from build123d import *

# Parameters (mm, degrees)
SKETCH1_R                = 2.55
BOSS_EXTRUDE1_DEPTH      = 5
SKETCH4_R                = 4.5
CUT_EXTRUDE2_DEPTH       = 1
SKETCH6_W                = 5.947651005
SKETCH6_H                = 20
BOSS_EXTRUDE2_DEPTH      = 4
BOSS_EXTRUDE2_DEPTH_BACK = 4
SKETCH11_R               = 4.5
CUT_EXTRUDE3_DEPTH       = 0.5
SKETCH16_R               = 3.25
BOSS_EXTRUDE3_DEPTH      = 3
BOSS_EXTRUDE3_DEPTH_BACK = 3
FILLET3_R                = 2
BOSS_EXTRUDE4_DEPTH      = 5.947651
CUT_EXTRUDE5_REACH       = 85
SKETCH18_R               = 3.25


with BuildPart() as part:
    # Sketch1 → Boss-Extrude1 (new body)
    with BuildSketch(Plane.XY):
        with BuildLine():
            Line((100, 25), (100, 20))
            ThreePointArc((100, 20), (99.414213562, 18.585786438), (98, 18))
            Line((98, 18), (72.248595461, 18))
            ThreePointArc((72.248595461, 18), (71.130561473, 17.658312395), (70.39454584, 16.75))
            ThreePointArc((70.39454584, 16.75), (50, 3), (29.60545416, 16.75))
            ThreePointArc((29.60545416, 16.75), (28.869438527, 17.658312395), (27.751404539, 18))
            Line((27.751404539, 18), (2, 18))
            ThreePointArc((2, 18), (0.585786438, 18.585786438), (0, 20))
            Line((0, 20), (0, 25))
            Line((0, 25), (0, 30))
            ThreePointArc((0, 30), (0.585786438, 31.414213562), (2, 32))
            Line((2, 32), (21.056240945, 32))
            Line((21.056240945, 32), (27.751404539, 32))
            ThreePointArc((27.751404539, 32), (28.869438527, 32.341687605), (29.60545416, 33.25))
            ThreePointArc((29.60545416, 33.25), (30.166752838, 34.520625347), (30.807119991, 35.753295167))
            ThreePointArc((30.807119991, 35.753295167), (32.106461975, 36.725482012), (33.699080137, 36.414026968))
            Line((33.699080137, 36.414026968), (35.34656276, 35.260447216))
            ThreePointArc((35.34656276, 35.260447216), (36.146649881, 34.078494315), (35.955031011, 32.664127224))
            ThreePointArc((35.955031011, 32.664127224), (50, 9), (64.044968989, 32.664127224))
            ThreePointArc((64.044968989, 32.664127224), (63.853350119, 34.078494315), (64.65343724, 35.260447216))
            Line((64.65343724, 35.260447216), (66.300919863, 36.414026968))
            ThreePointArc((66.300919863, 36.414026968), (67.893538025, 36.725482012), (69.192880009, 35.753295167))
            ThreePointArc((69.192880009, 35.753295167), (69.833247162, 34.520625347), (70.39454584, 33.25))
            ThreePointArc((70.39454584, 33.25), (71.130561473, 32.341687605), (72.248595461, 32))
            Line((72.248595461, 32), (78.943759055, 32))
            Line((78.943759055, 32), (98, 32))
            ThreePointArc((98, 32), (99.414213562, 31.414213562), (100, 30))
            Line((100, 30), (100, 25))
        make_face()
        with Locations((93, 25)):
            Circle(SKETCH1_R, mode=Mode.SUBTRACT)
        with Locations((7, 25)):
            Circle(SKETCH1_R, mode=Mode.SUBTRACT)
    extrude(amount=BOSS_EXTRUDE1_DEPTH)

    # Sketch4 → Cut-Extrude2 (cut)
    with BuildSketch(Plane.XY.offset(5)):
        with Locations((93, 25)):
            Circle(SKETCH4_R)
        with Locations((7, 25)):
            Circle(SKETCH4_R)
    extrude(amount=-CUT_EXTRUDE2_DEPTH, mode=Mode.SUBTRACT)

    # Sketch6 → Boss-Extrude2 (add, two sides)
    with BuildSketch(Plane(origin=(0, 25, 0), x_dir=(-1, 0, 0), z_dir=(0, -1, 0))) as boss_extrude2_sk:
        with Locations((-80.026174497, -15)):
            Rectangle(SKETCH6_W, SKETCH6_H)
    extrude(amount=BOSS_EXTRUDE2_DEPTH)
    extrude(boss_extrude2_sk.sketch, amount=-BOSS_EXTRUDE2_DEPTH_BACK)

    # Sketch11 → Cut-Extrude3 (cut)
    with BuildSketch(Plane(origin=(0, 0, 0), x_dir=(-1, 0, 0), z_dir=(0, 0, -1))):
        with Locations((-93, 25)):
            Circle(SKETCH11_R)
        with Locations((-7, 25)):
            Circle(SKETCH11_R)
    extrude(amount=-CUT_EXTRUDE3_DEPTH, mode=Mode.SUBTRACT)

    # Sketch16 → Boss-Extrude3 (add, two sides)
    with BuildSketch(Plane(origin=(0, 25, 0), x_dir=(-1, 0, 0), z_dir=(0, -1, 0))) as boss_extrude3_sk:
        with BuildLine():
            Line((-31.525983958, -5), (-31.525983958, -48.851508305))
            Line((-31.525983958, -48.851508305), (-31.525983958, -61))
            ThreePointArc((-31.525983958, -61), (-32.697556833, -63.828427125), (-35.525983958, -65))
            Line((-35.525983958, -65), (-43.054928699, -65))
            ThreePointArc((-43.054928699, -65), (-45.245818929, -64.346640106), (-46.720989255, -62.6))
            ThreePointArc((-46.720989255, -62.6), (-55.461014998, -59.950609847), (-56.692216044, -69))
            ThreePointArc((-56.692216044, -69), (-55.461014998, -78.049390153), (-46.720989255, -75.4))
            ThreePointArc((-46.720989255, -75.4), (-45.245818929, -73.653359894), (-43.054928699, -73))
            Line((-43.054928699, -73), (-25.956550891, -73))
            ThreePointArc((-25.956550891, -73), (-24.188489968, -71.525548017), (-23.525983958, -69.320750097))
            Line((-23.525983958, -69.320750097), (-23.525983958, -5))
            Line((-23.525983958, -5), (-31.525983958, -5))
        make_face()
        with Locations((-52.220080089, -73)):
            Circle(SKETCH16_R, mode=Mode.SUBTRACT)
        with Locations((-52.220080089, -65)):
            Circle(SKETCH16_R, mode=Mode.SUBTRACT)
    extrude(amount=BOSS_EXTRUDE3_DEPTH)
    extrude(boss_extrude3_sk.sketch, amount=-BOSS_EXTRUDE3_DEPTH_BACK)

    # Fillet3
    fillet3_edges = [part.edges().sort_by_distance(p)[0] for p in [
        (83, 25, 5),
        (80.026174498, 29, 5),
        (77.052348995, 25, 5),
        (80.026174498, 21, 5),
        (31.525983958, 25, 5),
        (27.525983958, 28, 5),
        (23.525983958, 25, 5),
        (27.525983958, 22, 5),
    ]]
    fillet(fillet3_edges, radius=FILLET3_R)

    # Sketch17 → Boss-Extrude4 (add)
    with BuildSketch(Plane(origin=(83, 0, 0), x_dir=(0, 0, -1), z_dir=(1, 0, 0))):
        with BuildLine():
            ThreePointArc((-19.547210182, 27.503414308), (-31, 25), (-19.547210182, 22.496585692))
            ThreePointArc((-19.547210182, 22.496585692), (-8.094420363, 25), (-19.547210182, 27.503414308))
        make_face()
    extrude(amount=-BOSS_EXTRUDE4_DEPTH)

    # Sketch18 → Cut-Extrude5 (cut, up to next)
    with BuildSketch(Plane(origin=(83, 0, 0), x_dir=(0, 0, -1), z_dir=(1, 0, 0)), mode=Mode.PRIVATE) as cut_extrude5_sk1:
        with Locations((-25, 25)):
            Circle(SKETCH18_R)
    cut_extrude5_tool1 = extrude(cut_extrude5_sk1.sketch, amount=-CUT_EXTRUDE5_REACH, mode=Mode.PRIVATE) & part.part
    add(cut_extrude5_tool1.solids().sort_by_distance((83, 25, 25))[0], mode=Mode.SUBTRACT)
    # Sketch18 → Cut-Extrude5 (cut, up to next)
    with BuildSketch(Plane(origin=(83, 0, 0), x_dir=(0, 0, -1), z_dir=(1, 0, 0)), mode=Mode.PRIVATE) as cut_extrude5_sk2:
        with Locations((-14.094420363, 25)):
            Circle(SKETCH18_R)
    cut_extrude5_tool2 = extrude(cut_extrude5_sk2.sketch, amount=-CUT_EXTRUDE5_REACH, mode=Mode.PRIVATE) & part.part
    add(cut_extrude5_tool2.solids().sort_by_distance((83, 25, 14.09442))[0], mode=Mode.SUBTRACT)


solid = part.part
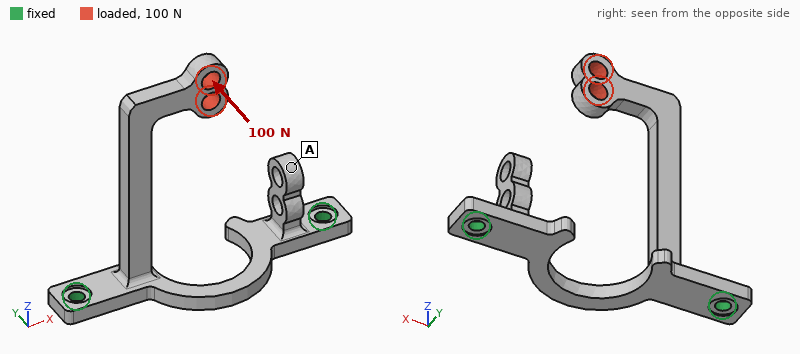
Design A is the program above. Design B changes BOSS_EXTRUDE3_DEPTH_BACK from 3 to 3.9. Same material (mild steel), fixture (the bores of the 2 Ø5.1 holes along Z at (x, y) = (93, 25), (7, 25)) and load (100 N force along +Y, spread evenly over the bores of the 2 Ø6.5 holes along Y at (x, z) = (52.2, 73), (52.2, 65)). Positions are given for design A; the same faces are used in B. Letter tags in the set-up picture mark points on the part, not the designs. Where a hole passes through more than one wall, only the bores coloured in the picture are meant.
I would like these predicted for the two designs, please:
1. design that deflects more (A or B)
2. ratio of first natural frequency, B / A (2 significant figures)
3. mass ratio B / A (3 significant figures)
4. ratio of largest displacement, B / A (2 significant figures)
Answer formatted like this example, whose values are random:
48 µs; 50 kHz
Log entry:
A; 1.0; 1.06; 0.78
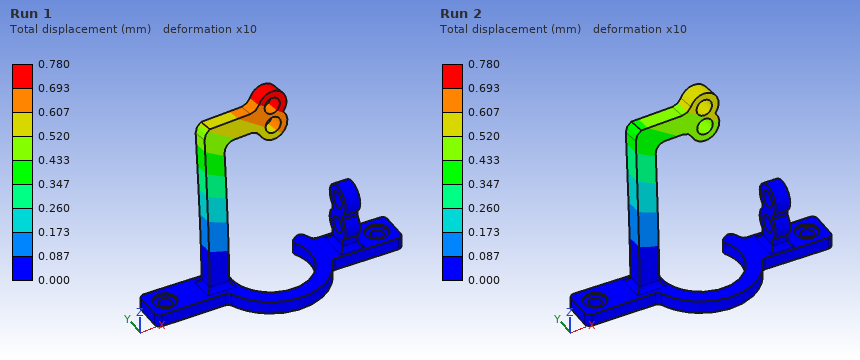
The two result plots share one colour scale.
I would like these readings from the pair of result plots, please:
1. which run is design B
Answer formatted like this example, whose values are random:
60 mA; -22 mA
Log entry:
Run 2
